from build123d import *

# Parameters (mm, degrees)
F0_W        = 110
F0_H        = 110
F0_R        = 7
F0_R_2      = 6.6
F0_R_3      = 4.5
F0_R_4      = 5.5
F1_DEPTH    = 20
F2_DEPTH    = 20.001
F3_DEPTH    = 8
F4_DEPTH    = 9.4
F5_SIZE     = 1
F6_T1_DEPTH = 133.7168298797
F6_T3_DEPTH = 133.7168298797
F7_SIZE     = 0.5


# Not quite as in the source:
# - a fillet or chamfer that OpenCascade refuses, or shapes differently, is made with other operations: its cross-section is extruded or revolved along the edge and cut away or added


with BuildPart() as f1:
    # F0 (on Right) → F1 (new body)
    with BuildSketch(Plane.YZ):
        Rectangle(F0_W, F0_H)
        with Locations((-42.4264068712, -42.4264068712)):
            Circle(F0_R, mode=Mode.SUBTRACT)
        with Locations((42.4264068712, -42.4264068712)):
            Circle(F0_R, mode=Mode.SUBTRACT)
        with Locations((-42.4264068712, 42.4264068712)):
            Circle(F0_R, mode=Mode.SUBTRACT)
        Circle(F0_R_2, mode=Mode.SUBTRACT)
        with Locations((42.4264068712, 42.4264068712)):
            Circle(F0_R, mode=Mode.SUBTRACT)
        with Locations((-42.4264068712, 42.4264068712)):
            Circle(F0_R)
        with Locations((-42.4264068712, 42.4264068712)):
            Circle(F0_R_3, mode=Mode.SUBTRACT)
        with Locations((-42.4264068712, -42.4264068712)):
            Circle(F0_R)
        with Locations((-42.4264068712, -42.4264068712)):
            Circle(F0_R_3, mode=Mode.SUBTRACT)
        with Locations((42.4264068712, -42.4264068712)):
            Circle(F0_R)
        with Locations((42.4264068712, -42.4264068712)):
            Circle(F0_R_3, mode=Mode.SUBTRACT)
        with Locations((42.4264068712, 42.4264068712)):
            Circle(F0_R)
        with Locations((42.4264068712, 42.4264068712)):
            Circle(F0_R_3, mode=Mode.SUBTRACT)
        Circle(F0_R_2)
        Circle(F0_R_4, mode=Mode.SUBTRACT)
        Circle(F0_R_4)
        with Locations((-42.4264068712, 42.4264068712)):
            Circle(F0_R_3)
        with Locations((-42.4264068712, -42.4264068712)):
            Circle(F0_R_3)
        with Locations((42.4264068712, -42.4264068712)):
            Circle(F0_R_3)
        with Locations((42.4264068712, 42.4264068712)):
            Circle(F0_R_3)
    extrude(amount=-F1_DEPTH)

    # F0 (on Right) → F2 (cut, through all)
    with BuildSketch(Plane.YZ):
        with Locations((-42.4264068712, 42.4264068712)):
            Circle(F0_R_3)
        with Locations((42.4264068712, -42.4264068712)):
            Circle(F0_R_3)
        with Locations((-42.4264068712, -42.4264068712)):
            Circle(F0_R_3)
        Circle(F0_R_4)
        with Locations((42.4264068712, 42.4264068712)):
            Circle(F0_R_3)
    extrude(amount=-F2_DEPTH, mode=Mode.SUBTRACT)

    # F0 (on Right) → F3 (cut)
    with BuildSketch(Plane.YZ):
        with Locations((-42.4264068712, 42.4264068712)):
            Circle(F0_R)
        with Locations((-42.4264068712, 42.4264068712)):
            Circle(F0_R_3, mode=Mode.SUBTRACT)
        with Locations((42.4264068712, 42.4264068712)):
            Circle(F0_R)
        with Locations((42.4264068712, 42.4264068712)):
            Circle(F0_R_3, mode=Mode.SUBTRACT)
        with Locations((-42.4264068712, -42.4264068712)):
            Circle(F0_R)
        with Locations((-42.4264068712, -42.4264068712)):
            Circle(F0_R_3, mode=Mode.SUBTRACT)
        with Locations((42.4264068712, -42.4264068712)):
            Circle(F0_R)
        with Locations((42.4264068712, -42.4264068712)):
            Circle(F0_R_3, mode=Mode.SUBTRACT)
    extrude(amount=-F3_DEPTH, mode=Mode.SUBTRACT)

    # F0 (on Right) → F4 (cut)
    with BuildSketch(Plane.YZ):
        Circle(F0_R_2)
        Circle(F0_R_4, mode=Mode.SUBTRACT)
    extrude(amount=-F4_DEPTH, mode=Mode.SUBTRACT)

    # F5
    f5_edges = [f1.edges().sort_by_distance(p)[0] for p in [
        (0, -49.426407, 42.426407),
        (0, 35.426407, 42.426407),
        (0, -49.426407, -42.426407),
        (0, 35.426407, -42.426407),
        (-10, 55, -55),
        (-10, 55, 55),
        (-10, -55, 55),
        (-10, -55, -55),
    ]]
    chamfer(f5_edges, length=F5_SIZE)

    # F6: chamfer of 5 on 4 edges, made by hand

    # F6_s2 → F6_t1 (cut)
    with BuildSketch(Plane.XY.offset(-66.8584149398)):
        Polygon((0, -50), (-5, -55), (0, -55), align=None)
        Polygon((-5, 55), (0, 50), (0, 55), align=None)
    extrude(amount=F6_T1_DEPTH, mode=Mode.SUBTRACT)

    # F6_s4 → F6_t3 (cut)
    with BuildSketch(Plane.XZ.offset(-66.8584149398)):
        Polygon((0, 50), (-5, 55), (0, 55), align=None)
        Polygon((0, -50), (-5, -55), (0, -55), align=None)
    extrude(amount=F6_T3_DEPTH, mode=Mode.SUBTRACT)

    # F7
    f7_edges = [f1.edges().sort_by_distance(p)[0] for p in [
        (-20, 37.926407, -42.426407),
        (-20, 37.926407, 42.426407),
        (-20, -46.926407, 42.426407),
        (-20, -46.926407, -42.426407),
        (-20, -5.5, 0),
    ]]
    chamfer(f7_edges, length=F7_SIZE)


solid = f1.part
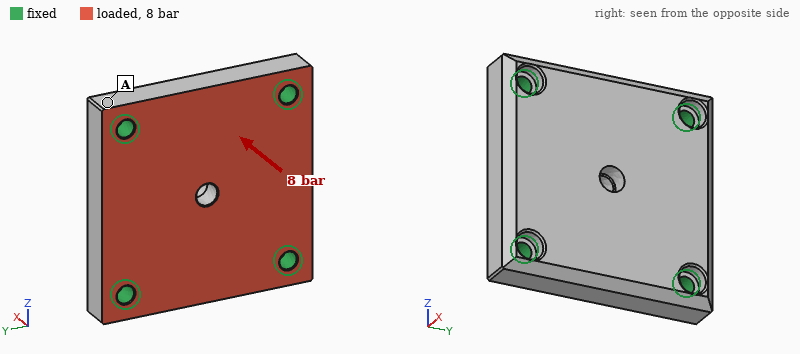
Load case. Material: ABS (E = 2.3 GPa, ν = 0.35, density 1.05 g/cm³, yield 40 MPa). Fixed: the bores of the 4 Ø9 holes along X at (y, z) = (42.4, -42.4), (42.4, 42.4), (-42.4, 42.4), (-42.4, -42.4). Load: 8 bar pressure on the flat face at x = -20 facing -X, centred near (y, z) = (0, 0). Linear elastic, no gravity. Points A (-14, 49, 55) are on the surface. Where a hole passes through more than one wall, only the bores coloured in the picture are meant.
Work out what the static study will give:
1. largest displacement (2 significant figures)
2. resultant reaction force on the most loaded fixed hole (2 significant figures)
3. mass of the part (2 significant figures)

0.36 mm
2.5 kN
240 g
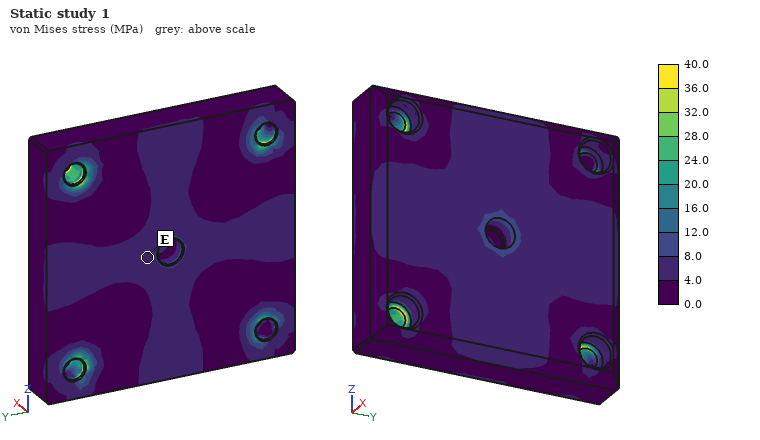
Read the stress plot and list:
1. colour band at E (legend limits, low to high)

4.0 to 8.0 MPa
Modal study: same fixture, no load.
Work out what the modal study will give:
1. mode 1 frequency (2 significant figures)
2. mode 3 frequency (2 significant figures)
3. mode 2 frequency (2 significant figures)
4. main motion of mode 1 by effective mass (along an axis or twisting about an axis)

2000 Hz
3000 Hz
3000 Hz
along X
